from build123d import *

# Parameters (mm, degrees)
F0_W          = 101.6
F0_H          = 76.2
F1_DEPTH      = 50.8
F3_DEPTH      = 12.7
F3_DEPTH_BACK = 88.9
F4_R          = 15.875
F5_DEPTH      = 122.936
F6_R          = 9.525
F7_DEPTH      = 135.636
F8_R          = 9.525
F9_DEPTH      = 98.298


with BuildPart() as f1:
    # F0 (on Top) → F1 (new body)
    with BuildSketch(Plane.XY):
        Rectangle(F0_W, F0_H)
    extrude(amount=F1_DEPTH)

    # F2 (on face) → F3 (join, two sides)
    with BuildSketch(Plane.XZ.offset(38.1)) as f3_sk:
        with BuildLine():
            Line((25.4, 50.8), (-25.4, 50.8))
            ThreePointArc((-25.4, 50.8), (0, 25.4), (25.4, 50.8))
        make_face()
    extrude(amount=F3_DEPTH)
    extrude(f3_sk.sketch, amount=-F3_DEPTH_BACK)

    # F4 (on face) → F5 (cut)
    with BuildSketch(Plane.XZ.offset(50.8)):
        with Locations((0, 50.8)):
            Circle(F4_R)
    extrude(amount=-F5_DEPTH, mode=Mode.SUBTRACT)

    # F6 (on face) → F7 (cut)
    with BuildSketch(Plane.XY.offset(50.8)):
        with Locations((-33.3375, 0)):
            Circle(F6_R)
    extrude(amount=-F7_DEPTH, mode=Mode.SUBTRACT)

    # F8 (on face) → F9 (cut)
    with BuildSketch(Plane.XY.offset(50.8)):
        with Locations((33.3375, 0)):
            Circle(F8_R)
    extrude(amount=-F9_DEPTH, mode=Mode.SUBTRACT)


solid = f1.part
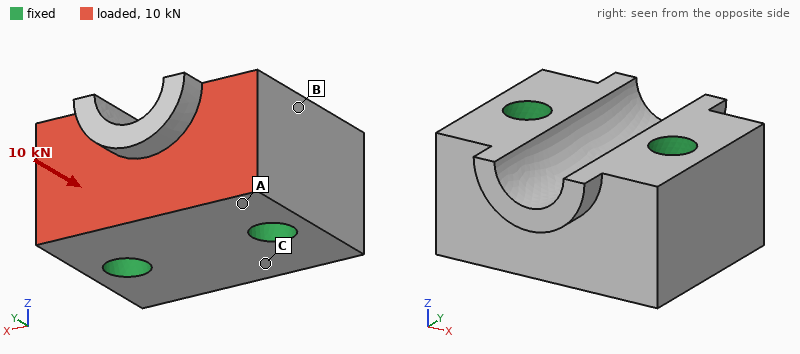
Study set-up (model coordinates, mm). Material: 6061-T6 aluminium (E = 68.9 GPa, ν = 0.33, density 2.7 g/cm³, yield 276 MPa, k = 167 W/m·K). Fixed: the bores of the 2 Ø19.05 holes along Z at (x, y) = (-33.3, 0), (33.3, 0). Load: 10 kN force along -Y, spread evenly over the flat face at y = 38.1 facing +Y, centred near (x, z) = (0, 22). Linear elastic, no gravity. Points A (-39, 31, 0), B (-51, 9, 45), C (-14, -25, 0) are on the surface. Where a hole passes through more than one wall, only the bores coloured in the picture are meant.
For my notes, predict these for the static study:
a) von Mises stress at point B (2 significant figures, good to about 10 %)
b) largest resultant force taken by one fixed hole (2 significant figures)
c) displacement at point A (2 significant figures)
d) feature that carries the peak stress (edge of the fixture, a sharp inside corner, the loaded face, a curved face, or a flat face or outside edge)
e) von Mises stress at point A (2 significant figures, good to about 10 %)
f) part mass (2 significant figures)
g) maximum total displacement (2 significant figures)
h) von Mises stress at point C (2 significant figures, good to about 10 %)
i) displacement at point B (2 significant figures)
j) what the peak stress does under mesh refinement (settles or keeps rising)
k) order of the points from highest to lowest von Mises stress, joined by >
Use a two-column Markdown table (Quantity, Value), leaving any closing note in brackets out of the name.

| Quantity | Value |
|---|---|
| von Mises stress at point B | 1.4 MPa |
| largest resultant force taken by one fixed hole | 5.0 kN |
| displacement at point A | 1.2 µm |
| feature that carries the peak stress | edge of the fixture |
| von Mises stress at point A | 2.5 MPa |
| part mass | 940 g |
| maximum total displacement | 1.8 µm |
| von Mises stress at point C | 0.60 MPa |
| displacement at point B | 0.38 µm |
| what the peak stress does under mesh refinement | keeps rising |
| order of the points from highest to lowest von Mises stress, joined by > | A > B > C |
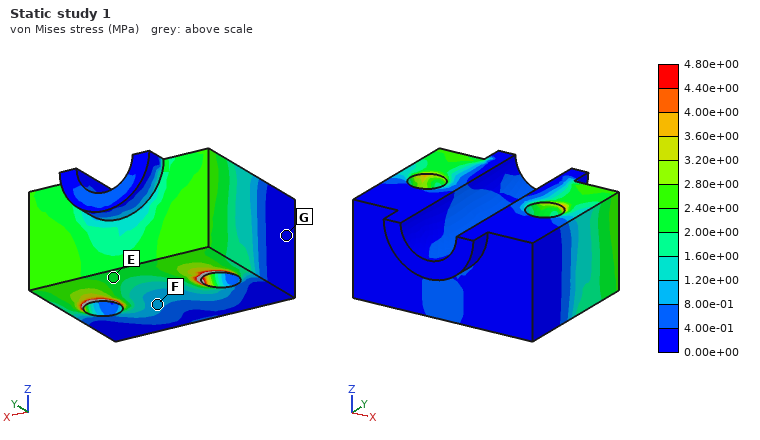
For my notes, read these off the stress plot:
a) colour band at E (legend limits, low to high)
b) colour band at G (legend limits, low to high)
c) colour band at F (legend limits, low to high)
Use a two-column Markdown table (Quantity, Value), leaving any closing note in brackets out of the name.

| Quantity | Value |
|---|---|
| colour band at E | 2.00e+00 to 2.40e+00 MPa |
| colour band at G | 0.00e+00 to 4.00e-01 MPa |
| colour band at F | 8.00e-01 to 1.20e+00 MPa |
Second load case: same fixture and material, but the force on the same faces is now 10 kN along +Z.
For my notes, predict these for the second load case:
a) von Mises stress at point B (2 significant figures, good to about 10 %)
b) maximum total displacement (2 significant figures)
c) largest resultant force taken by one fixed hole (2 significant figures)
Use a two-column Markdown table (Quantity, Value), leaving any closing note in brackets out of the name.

| Quantity | Value |
|---|---|
| von Mises stress at point B | 2.9 MPa |
| maximum total displacement | 7.1 µm |
| largest resultant force taken by one fixed hole | 5.0 kN |
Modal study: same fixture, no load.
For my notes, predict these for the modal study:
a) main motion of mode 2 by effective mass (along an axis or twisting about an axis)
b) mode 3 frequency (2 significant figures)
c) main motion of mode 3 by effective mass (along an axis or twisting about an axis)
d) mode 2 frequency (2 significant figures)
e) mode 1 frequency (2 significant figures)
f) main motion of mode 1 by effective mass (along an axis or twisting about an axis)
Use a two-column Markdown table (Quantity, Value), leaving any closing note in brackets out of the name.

| Quantity | Value |
|---|---|
| main motion of mode 2 by effective mass | along Z |
| mode 3 frequency | 17 kHz |
| main motion of mode 3 by effective mass | twisting about Z |
| mode 2 frequency | 15 kHz |
| mode 1 frequency | 15 kHz |
| main motion of mode 1 by effective mass | twisting about X |
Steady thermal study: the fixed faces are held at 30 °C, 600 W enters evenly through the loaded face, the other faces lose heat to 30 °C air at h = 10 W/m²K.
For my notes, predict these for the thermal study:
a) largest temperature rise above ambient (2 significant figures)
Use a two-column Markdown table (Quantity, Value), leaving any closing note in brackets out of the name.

| Quantity | Value |
|---|---|
| largest temperature rise above ambient | 29 K |
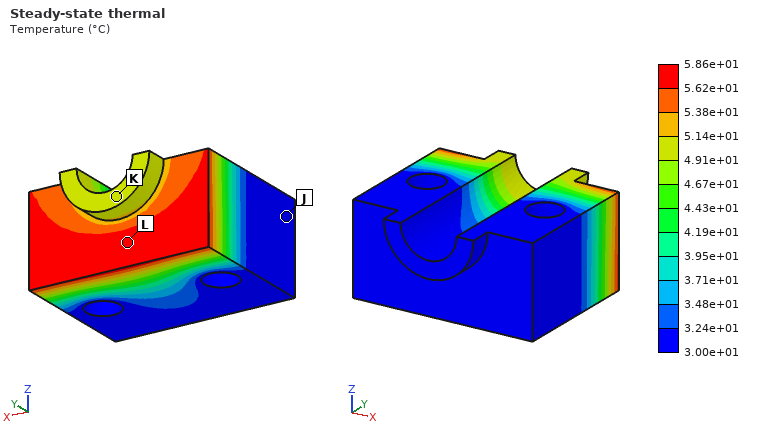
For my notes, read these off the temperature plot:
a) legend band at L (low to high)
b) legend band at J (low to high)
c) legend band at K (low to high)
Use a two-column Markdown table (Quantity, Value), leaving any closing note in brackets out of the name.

| Quantity | Value |
|---|---|
| legend band at L | 5.62e+01 to 5.86e+01 °C |
| legend band at J | 3.00e+01 to 3.24e+01 °C |
| legend band at K | 4.91e+01 to 5.14e+01 °C |
